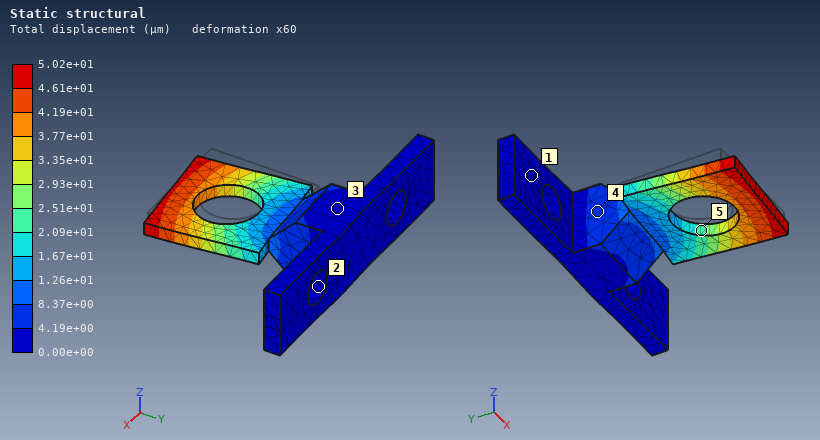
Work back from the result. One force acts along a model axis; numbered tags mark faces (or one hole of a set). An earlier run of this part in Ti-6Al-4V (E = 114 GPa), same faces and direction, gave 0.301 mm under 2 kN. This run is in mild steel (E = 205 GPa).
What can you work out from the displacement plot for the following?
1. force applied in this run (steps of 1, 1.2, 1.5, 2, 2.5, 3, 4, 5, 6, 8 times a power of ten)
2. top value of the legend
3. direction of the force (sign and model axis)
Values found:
600 N
5.02e+01 µm
+X
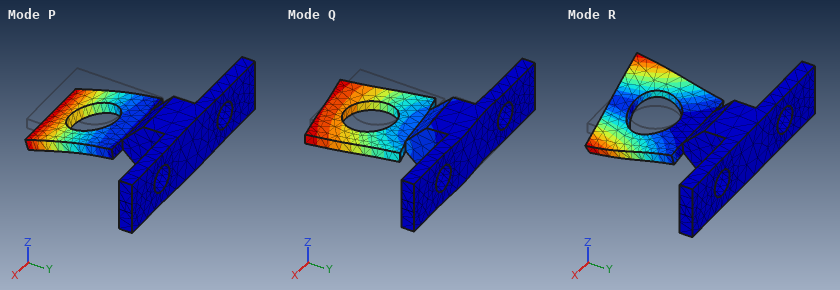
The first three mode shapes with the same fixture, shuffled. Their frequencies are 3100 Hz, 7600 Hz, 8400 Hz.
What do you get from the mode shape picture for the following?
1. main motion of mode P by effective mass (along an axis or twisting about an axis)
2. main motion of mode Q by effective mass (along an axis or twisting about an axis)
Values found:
along Z
along X
